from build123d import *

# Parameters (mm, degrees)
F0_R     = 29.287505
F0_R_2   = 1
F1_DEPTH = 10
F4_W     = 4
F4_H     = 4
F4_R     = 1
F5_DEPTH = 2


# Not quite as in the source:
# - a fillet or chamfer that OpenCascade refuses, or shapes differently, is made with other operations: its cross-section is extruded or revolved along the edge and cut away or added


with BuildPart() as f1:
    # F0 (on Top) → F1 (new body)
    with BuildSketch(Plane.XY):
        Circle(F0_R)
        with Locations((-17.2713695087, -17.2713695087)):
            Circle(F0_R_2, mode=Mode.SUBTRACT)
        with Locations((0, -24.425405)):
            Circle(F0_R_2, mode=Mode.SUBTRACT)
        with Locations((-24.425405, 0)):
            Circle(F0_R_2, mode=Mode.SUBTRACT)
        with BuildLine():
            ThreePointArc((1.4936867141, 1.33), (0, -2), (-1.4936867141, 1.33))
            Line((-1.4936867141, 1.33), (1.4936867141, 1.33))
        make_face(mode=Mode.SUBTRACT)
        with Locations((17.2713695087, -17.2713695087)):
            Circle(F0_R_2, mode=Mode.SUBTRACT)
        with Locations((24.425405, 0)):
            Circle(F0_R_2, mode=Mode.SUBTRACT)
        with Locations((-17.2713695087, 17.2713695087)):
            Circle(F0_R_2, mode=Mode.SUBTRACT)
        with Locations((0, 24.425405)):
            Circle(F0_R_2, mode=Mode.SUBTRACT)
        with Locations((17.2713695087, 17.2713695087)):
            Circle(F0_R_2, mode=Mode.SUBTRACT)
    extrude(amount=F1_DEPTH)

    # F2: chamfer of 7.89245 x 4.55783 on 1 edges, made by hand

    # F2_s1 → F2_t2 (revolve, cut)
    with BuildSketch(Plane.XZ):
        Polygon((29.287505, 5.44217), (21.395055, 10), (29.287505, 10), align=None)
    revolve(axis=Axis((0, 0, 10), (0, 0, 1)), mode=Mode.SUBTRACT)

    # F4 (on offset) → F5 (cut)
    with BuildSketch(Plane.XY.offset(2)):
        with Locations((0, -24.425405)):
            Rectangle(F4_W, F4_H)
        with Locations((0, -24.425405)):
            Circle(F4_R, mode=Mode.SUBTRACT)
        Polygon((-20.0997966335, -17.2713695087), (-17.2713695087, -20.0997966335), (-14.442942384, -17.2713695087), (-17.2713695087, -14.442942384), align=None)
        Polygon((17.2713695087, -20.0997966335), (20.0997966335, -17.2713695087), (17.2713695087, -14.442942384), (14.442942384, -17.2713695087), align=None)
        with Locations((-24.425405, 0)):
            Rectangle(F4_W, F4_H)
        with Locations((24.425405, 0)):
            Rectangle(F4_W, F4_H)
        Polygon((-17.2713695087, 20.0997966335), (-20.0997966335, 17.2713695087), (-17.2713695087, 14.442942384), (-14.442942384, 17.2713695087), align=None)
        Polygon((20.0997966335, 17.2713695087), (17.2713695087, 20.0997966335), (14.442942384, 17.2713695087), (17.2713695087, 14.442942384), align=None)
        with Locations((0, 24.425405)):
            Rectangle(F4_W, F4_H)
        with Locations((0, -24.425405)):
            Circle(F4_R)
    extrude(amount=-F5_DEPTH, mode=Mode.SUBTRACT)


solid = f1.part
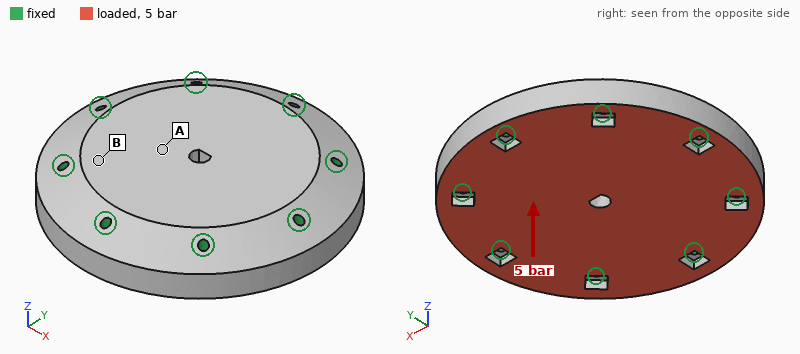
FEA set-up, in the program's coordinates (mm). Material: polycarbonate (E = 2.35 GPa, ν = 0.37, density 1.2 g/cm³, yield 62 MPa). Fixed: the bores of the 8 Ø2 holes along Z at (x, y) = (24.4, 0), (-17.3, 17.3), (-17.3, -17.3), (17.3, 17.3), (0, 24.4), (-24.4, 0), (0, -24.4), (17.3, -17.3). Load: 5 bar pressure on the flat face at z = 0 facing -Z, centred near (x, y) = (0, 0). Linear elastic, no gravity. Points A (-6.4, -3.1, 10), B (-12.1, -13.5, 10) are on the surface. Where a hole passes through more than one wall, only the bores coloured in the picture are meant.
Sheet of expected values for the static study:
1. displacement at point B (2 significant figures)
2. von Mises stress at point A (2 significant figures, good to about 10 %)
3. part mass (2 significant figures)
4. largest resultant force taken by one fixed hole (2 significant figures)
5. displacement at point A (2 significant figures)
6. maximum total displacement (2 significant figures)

21 µm
2.3 MPa
28 g
160 N
38 µm
45 µm
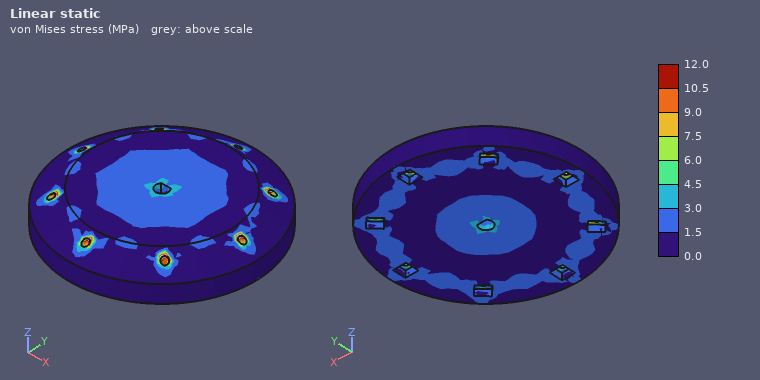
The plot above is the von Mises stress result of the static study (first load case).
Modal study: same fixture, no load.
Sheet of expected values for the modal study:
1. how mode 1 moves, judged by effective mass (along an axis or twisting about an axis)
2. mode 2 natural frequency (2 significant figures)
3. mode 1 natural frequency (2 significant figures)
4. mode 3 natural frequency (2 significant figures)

along Z
11 kHz
5800 Hz
11 kHz
